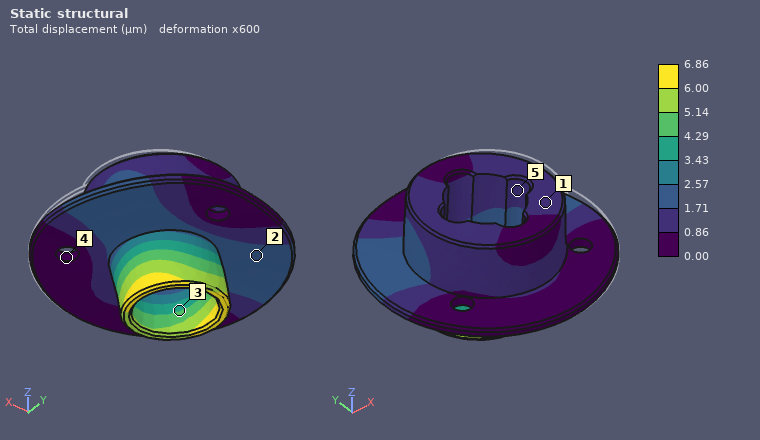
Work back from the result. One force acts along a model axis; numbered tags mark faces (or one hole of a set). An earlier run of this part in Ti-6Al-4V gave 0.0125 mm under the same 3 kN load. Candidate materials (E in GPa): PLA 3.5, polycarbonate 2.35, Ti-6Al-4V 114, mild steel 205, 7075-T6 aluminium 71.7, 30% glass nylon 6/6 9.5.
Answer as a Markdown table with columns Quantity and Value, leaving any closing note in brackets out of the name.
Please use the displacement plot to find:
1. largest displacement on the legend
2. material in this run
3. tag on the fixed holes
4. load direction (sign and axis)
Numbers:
| Quantity | Value |
|---|---|
| largest displacement on the legend | 6.86 µm |
| material in this run | mild steel |
| tag on the fixed holes | 4 |
| load direction | -X |
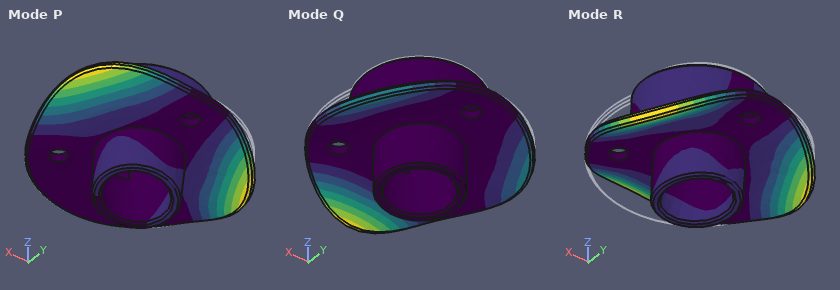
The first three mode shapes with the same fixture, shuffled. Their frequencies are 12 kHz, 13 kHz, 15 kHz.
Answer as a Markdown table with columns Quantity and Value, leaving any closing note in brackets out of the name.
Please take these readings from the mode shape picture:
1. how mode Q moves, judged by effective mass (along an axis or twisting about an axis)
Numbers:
| Quantity | Value |
|---|---|
| how mode Q moves, judged by effective mass | along Z |
